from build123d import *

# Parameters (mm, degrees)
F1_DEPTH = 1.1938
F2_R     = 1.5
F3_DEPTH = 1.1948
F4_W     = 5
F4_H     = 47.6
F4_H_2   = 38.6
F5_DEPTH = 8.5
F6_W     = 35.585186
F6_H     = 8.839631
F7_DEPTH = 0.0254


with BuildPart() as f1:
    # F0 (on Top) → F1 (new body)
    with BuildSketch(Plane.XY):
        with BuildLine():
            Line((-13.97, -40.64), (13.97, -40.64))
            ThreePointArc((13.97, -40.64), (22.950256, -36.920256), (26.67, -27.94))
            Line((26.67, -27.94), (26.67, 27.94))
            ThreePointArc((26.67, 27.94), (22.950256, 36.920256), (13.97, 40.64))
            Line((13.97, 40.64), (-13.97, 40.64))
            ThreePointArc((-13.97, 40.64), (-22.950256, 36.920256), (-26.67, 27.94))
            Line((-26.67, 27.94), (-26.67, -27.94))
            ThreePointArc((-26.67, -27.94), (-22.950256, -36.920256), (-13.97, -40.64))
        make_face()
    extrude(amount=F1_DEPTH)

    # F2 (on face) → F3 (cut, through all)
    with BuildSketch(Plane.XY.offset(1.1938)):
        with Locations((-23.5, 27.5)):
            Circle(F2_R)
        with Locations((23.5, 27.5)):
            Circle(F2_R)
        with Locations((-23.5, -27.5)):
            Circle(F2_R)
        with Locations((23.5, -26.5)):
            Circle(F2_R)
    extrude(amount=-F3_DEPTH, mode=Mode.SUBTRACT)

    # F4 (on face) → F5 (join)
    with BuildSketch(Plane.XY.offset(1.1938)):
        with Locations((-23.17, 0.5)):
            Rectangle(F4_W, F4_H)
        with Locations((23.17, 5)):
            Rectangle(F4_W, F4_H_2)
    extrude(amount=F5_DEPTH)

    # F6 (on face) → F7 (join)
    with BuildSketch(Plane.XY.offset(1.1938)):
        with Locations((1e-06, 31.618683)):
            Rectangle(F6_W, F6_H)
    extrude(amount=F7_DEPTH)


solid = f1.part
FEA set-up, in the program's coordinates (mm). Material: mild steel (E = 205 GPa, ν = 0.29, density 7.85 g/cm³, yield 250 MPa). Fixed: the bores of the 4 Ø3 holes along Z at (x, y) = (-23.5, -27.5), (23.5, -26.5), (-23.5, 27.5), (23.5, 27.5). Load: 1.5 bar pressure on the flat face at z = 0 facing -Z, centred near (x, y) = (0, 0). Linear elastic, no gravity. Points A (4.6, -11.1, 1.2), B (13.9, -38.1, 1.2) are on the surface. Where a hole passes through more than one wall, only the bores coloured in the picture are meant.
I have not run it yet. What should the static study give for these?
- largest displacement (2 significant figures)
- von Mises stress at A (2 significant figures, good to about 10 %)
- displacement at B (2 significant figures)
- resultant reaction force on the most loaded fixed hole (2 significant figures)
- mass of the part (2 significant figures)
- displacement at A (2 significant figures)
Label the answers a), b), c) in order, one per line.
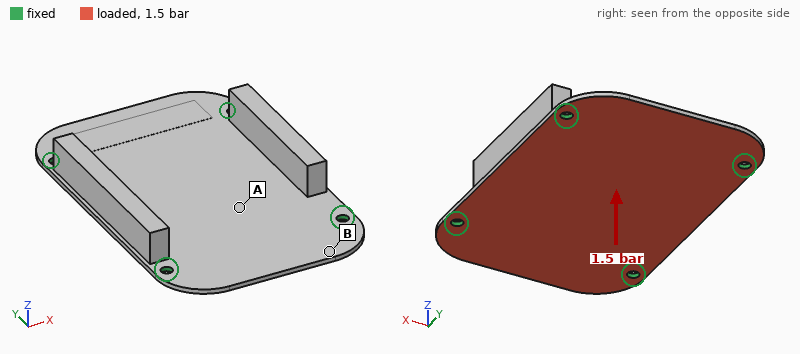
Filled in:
a) 0.10 mm
b) 51 MPa
c) 0.056 mm
d) 180 N
e) 68 g
f) 0.090 mm
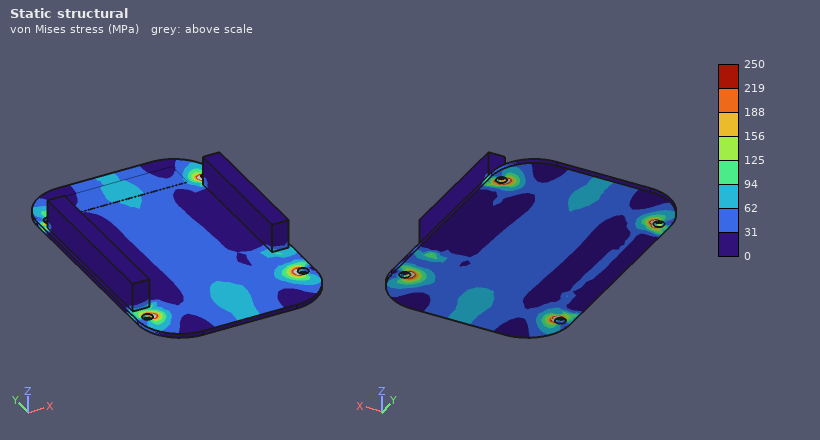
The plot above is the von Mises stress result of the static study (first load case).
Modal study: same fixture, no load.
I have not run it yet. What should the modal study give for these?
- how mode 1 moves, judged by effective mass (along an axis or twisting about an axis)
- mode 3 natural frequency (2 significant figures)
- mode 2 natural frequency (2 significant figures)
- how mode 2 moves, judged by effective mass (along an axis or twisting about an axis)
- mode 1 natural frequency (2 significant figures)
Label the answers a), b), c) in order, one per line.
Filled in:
a) along Z
b) 2800 Hz
c) 2600 Hz
d) twisting about X
e) 2300 Hz
